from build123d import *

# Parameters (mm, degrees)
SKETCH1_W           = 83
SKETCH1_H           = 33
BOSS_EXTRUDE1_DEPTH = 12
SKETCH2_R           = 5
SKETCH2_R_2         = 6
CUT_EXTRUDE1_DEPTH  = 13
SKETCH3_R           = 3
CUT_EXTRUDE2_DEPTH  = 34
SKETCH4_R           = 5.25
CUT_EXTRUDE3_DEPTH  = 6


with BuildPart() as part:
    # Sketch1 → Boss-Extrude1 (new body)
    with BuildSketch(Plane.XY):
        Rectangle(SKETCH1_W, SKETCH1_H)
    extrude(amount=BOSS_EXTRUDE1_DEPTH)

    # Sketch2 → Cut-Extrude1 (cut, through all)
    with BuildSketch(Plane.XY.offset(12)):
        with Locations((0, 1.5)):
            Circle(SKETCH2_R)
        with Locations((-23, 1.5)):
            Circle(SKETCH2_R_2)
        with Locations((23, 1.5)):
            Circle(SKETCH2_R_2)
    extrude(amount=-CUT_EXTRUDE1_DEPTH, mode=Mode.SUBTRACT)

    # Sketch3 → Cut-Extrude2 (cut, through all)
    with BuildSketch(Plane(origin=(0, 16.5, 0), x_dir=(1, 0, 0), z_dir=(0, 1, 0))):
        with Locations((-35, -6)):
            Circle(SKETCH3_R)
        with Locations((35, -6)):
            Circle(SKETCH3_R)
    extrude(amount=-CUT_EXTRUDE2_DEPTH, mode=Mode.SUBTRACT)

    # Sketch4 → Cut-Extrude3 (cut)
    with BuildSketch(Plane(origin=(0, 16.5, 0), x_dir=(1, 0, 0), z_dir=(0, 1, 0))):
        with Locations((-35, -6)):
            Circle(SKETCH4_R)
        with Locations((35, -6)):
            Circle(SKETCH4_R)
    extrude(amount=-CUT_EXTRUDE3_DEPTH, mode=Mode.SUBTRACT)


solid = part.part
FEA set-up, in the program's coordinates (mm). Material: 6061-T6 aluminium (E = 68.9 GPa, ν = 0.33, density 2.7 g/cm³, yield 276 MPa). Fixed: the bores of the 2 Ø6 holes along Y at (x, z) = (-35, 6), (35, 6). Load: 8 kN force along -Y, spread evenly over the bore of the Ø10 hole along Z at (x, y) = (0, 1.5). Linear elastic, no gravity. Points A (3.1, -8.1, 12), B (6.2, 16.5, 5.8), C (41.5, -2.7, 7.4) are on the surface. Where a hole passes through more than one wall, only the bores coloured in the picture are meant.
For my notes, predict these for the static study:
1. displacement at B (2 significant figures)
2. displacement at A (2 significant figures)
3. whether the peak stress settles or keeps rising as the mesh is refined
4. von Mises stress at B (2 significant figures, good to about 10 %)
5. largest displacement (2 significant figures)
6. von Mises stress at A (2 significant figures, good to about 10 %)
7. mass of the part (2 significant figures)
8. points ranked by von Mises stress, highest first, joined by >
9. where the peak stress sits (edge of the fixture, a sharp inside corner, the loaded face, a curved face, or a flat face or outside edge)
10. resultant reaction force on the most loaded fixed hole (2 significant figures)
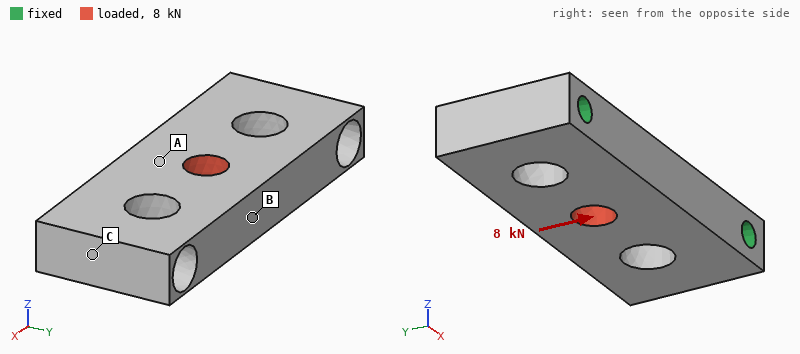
29 µm
32 µm
keeps rising
38 MPa
34 µm
16 MPa
72 g
B > A > C
edge of the fixture
4.2 kN
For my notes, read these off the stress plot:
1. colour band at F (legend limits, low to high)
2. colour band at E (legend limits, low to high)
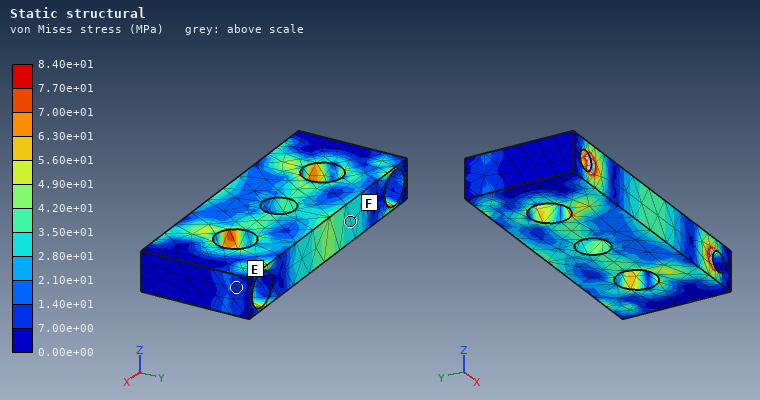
2.80e+01 to 3.50e+01 MPa
7.00e+00 to 1.40e+01 MPa
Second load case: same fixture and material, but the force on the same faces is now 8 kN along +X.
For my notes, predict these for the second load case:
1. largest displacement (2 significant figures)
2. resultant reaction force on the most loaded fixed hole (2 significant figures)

9.9 µm
4.0 kN
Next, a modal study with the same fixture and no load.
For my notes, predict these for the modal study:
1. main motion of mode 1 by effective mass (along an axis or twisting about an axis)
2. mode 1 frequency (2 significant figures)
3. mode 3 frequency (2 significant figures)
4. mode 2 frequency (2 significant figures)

along Z
9500 Hz
14 kHz
14 kHz
